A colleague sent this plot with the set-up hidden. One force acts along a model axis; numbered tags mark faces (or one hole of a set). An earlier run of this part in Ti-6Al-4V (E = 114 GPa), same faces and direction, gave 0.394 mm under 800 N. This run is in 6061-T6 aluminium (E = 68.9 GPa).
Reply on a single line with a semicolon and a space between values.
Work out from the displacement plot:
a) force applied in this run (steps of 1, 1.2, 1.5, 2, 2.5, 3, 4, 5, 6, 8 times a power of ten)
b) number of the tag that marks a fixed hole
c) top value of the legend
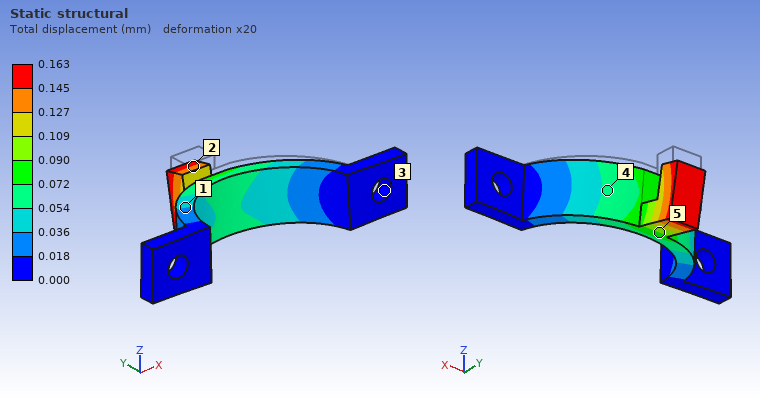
200 N; 3; 0.163 mm
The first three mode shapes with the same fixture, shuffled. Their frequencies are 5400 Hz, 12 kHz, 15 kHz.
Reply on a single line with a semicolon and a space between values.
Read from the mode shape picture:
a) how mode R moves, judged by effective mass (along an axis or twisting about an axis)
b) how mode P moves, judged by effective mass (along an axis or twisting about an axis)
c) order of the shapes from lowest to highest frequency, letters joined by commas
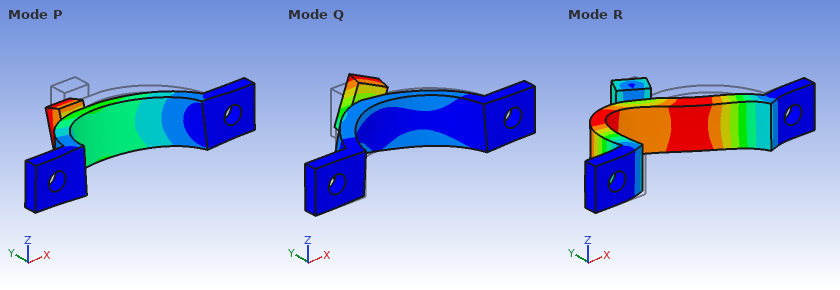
along X; along Z; P, R, Q
